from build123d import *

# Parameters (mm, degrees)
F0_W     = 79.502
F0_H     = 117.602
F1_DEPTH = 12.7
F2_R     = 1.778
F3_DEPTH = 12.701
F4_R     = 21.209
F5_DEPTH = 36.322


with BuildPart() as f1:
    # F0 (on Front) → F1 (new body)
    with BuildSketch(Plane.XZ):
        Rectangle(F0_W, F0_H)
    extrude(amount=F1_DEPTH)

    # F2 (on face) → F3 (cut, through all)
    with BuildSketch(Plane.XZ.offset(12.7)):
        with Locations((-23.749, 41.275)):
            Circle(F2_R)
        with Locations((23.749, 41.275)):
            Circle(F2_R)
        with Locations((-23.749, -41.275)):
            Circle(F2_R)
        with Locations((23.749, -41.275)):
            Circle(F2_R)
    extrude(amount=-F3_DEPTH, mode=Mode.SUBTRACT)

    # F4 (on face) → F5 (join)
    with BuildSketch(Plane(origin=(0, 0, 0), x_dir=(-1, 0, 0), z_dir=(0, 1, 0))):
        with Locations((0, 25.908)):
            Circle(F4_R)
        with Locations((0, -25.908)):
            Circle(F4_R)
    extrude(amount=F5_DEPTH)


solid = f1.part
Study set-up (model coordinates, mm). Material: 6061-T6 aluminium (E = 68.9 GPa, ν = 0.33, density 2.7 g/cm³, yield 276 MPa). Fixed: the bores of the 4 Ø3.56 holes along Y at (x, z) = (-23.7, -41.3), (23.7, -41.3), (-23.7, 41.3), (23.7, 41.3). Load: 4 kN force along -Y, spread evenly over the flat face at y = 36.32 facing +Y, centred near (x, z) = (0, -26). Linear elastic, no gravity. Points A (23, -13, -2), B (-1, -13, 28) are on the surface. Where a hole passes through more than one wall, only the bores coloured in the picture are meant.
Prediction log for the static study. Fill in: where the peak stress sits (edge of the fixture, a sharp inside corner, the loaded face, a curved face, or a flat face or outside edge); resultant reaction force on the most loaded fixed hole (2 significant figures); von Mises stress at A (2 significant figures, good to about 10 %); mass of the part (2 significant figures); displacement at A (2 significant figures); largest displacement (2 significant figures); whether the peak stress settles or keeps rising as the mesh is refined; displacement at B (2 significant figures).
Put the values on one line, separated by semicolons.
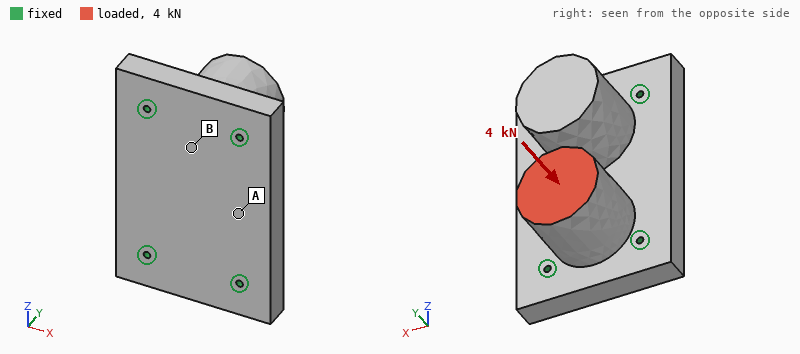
edge of the fixture; 1.7 kN; 6.1 MPa; 600 g; 9.1 µm; 16 µm; keeps rising; 4.0 µm
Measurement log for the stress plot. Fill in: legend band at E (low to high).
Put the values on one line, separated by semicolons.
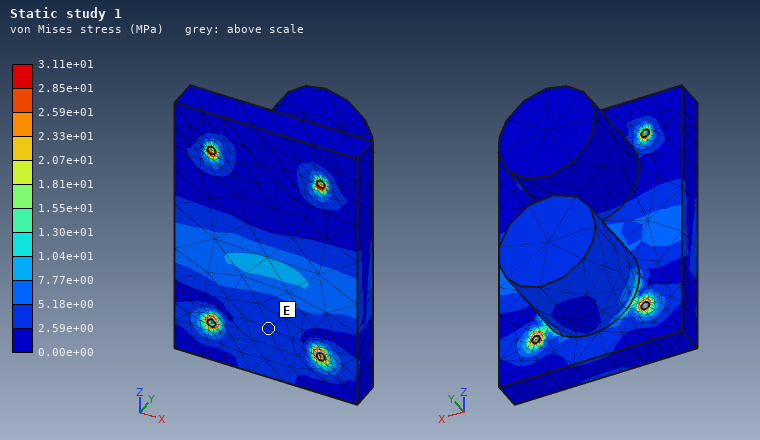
2.59e+00 to 5.18e+00 MPa
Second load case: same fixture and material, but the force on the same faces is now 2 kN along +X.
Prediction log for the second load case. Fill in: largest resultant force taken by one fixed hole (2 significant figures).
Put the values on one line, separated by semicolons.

1.8 kN
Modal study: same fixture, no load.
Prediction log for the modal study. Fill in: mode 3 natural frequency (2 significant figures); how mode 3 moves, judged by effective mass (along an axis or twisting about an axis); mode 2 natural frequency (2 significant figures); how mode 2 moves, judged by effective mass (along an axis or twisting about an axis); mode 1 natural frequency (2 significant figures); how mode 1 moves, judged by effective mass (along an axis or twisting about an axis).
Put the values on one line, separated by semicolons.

7900 Hz; along Z; 6600 Hz; along X; 3800 Hz; along Y
